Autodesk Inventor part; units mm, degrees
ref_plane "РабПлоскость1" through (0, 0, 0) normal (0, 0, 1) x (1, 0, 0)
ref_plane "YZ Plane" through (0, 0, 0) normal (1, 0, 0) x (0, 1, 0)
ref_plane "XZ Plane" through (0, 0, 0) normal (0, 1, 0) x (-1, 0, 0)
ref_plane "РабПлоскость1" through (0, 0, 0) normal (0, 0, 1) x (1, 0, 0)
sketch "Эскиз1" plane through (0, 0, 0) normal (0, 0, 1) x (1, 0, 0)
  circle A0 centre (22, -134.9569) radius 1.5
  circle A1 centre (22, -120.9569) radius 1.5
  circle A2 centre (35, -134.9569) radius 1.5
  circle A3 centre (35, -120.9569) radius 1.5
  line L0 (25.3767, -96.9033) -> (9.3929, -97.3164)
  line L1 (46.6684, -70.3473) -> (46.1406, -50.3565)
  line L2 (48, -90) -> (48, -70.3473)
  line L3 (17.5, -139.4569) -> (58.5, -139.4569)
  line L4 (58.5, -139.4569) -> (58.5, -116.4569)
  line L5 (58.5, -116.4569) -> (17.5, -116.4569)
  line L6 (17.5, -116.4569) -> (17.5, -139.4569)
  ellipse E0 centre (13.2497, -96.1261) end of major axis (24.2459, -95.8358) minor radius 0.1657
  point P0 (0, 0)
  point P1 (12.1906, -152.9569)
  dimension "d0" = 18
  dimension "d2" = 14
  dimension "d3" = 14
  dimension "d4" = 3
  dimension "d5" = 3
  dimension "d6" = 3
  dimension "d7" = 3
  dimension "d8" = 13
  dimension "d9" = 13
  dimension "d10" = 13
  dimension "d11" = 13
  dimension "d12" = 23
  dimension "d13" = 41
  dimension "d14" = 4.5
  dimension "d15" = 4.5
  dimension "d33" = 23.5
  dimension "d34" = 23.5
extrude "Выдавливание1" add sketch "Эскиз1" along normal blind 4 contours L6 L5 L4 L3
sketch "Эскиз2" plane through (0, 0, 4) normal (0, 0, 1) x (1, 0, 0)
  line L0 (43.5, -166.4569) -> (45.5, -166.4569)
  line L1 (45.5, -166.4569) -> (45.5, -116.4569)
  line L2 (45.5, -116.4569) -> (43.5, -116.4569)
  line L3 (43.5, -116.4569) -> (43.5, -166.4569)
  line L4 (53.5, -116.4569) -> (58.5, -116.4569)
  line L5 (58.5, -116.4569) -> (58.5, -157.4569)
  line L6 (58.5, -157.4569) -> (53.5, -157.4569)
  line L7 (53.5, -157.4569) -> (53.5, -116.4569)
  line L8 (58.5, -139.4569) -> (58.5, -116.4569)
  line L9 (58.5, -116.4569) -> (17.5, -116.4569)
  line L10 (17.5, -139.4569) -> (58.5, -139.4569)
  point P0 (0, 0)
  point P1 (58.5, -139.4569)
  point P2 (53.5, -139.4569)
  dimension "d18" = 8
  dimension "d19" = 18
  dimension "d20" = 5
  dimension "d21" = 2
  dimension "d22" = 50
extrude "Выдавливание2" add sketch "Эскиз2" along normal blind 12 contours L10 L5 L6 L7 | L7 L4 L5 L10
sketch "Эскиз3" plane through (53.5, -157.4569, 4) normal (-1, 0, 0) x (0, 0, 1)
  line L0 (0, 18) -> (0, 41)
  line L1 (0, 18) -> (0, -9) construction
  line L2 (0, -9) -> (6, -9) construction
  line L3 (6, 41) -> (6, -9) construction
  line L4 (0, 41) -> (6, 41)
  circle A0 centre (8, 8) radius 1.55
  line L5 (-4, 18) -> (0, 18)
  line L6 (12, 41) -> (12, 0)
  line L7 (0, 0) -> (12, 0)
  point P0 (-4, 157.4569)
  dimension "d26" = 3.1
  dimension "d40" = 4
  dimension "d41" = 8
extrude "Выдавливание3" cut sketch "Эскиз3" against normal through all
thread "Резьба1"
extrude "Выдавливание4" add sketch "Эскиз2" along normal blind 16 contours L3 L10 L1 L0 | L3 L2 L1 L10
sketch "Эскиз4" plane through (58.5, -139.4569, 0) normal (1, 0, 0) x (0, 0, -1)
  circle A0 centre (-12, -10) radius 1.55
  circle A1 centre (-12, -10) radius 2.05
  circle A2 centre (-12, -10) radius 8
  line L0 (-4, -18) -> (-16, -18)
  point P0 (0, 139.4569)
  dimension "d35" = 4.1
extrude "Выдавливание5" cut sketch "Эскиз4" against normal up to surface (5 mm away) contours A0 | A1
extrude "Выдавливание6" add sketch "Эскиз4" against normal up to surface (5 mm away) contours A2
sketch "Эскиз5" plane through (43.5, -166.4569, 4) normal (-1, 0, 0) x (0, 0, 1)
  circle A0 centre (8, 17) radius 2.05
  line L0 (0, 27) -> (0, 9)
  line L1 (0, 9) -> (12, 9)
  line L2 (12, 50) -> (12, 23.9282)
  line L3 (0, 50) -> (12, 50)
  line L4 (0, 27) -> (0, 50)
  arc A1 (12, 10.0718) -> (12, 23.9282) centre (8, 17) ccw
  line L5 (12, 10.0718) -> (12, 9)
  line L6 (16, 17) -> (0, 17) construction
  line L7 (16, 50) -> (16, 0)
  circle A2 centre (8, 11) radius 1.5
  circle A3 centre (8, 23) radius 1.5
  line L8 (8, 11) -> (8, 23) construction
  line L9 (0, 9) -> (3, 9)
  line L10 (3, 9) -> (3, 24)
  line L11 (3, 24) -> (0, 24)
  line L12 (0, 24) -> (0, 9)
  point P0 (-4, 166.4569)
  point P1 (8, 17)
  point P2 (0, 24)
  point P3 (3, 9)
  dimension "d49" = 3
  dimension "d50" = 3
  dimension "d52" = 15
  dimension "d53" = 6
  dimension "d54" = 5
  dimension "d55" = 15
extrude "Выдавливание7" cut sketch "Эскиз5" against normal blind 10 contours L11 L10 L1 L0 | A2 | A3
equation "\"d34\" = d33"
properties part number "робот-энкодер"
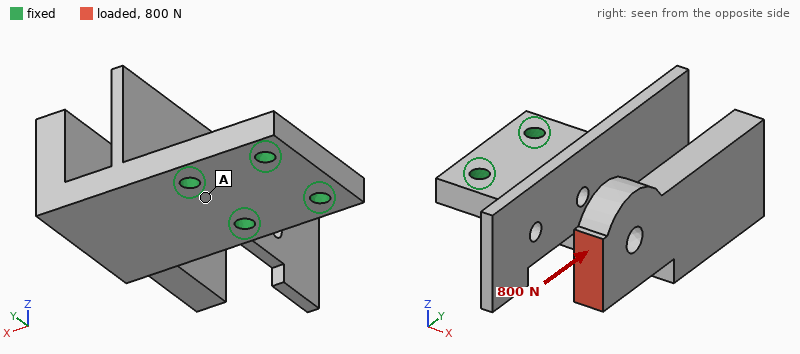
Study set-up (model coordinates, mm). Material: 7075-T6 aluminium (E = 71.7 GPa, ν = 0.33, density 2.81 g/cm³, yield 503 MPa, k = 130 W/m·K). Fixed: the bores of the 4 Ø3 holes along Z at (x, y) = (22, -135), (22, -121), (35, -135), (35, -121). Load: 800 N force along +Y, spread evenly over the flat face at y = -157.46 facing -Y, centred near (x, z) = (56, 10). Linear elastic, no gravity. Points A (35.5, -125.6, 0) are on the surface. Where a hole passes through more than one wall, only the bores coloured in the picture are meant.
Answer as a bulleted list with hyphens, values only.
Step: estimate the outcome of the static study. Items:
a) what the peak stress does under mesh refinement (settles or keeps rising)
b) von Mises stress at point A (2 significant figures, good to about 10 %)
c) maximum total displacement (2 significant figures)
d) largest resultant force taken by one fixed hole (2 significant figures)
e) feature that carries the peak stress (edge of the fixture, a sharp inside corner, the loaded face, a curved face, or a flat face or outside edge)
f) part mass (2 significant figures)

- keeps rising
- 16 MPa
- 0.20 mm
- 1.1 kN
- edge of the fixture
- 22 g
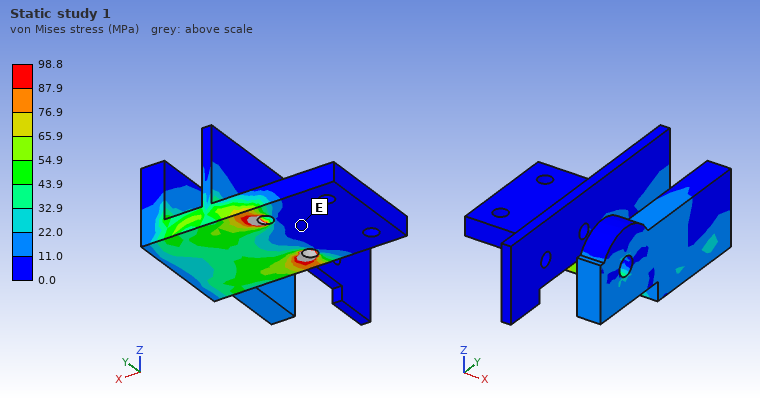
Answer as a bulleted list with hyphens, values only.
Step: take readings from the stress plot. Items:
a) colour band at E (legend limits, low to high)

- 0.0 to 11.0 MPa
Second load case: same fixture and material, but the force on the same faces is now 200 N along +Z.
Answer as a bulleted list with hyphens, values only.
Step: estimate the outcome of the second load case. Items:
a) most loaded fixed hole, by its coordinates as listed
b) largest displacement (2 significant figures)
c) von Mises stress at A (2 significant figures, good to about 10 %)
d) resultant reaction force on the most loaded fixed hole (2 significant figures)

- (35, -135)
- 0.28 mm
- 28 MPa
- 500 N
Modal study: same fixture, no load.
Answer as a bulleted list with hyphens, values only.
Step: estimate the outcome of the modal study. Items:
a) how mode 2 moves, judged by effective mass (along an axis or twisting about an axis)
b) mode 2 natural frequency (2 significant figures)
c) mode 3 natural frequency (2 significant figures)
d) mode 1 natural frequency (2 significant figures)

- along Z
- 2200 Hz
- 3500 Hz
- 1400 Hz
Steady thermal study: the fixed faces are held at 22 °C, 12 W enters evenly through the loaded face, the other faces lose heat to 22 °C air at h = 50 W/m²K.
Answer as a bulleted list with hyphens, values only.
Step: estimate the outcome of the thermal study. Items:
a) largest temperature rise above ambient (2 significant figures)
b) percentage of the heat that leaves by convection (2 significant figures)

- 52 K
- 26 %
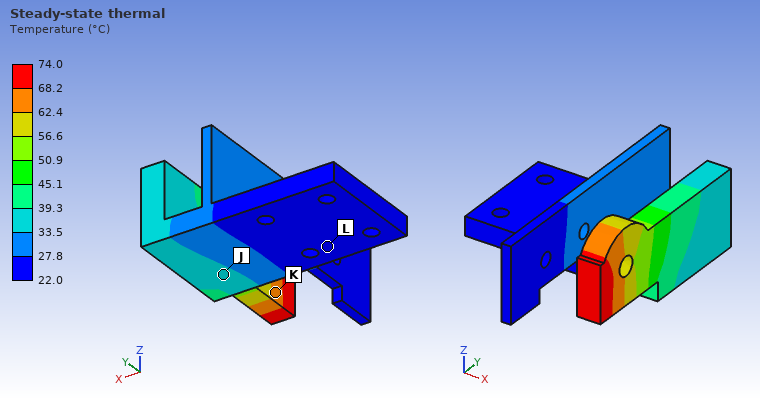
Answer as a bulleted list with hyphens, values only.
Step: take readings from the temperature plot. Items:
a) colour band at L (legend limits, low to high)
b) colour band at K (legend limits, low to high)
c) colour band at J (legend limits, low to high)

- 22.0 to 27.8 °C
- 62.4 to 68.2 °C
- 33.5 to 39.3 °C
